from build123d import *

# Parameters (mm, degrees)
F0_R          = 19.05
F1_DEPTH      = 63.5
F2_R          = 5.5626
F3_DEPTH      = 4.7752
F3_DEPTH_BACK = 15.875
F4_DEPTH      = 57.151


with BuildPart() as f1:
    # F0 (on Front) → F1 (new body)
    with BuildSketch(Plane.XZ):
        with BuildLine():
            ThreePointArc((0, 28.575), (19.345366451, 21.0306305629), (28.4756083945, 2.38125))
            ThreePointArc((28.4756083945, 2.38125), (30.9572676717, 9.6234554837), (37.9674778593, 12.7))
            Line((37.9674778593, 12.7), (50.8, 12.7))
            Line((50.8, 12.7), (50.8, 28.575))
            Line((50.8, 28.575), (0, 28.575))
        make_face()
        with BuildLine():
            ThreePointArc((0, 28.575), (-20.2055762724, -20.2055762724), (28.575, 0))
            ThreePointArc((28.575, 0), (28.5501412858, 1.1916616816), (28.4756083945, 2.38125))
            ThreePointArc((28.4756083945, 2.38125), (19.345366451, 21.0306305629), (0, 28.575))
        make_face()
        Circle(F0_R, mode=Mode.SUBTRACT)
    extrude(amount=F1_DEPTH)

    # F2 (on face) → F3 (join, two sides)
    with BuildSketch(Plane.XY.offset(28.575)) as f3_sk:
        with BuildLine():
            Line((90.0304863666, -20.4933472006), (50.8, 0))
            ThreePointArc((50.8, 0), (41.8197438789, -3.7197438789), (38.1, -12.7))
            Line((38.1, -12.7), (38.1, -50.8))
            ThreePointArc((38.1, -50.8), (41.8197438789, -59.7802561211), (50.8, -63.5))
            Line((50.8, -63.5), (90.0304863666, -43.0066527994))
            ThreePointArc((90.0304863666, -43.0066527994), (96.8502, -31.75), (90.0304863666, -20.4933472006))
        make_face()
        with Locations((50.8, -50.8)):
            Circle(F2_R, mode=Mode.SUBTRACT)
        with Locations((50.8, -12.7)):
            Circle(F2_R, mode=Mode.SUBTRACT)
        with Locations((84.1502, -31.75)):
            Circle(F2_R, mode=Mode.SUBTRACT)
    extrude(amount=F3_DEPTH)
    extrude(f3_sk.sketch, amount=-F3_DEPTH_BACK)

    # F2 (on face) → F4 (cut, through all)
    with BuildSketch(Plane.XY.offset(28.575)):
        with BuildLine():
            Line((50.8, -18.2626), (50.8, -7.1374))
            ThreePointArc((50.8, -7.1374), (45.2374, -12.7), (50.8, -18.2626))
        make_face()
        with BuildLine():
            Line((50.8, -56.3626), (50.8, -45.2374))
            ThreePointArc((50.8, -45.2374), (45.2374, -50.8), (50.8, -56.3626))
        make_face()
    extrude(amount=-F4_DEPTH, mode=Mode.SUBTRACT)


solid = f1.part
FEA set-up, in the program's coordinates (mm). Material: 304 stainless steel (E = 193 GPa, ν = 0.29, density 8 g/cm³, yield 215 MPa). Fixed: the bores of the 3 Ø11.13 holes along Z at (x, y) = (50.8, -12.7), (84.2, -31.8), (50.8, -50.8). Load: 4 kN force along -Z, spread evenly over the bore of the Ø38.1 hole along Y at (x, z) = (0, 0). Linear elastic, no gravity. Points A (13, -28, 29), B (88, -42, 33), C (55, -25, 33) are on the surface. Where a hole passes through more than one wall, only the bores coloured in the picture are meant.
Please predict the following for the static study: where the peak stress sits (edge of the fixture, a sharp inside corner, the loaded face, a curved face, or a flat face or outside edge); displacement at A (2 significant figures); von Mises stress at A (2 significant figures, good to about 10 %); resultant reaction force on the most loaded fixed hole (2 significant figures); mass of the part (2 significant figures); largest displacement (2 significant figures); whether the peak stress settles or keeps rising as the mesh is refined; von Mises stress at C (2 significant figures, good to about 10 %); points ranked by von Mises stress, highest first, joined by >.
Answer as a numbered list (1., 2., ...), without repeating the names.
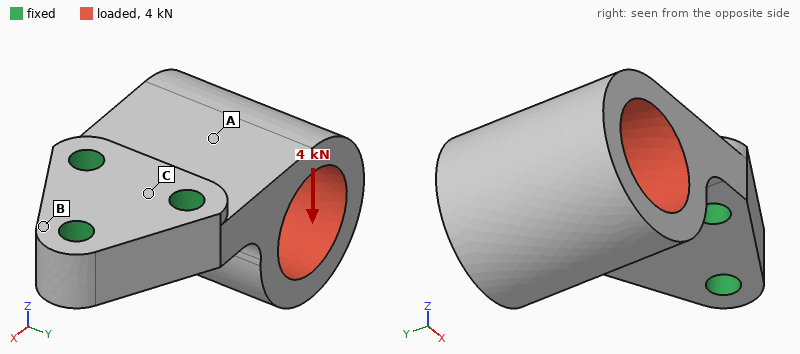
1. edge of the fixture
2. 19 µm
3. 20 MPa
4. 2.3 kN
5. 1.3 kg
6. 64 µm
7. keeps rising
8. 14 MPa
9. A > C > B
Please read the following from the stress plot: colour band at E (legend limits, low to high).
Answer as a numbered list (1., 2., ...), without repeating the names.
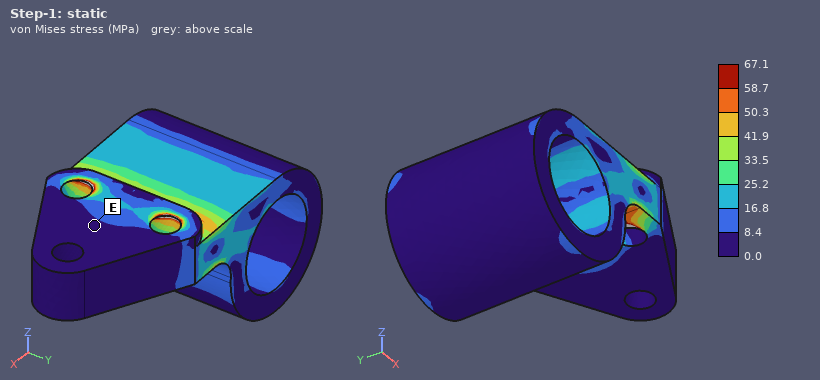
1. 0.0 to 8.4 MPa
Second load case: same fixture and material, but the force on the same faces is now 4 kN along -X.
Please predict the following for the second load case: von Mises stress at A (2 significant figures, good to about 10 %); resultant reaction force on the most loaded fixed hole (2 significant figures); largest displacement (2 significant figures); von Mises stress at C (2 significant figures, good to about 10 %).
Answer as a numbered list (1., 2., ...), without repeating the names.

1. 7.2 MPa
2. 1.9 kN
3. 39 µm
4. 5.2 MPa
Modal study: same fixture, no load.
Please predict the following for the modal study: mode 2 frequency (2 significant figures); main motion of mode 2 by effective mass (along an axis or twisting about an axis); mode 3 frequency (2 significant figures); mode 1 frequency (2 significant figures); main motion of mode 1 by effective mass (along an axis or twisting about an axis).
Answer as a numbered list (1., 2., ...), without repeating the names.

1. 3600 Hz
2. along Y
3. 5800 Hz
4. 1500 Hz
5. along Z
